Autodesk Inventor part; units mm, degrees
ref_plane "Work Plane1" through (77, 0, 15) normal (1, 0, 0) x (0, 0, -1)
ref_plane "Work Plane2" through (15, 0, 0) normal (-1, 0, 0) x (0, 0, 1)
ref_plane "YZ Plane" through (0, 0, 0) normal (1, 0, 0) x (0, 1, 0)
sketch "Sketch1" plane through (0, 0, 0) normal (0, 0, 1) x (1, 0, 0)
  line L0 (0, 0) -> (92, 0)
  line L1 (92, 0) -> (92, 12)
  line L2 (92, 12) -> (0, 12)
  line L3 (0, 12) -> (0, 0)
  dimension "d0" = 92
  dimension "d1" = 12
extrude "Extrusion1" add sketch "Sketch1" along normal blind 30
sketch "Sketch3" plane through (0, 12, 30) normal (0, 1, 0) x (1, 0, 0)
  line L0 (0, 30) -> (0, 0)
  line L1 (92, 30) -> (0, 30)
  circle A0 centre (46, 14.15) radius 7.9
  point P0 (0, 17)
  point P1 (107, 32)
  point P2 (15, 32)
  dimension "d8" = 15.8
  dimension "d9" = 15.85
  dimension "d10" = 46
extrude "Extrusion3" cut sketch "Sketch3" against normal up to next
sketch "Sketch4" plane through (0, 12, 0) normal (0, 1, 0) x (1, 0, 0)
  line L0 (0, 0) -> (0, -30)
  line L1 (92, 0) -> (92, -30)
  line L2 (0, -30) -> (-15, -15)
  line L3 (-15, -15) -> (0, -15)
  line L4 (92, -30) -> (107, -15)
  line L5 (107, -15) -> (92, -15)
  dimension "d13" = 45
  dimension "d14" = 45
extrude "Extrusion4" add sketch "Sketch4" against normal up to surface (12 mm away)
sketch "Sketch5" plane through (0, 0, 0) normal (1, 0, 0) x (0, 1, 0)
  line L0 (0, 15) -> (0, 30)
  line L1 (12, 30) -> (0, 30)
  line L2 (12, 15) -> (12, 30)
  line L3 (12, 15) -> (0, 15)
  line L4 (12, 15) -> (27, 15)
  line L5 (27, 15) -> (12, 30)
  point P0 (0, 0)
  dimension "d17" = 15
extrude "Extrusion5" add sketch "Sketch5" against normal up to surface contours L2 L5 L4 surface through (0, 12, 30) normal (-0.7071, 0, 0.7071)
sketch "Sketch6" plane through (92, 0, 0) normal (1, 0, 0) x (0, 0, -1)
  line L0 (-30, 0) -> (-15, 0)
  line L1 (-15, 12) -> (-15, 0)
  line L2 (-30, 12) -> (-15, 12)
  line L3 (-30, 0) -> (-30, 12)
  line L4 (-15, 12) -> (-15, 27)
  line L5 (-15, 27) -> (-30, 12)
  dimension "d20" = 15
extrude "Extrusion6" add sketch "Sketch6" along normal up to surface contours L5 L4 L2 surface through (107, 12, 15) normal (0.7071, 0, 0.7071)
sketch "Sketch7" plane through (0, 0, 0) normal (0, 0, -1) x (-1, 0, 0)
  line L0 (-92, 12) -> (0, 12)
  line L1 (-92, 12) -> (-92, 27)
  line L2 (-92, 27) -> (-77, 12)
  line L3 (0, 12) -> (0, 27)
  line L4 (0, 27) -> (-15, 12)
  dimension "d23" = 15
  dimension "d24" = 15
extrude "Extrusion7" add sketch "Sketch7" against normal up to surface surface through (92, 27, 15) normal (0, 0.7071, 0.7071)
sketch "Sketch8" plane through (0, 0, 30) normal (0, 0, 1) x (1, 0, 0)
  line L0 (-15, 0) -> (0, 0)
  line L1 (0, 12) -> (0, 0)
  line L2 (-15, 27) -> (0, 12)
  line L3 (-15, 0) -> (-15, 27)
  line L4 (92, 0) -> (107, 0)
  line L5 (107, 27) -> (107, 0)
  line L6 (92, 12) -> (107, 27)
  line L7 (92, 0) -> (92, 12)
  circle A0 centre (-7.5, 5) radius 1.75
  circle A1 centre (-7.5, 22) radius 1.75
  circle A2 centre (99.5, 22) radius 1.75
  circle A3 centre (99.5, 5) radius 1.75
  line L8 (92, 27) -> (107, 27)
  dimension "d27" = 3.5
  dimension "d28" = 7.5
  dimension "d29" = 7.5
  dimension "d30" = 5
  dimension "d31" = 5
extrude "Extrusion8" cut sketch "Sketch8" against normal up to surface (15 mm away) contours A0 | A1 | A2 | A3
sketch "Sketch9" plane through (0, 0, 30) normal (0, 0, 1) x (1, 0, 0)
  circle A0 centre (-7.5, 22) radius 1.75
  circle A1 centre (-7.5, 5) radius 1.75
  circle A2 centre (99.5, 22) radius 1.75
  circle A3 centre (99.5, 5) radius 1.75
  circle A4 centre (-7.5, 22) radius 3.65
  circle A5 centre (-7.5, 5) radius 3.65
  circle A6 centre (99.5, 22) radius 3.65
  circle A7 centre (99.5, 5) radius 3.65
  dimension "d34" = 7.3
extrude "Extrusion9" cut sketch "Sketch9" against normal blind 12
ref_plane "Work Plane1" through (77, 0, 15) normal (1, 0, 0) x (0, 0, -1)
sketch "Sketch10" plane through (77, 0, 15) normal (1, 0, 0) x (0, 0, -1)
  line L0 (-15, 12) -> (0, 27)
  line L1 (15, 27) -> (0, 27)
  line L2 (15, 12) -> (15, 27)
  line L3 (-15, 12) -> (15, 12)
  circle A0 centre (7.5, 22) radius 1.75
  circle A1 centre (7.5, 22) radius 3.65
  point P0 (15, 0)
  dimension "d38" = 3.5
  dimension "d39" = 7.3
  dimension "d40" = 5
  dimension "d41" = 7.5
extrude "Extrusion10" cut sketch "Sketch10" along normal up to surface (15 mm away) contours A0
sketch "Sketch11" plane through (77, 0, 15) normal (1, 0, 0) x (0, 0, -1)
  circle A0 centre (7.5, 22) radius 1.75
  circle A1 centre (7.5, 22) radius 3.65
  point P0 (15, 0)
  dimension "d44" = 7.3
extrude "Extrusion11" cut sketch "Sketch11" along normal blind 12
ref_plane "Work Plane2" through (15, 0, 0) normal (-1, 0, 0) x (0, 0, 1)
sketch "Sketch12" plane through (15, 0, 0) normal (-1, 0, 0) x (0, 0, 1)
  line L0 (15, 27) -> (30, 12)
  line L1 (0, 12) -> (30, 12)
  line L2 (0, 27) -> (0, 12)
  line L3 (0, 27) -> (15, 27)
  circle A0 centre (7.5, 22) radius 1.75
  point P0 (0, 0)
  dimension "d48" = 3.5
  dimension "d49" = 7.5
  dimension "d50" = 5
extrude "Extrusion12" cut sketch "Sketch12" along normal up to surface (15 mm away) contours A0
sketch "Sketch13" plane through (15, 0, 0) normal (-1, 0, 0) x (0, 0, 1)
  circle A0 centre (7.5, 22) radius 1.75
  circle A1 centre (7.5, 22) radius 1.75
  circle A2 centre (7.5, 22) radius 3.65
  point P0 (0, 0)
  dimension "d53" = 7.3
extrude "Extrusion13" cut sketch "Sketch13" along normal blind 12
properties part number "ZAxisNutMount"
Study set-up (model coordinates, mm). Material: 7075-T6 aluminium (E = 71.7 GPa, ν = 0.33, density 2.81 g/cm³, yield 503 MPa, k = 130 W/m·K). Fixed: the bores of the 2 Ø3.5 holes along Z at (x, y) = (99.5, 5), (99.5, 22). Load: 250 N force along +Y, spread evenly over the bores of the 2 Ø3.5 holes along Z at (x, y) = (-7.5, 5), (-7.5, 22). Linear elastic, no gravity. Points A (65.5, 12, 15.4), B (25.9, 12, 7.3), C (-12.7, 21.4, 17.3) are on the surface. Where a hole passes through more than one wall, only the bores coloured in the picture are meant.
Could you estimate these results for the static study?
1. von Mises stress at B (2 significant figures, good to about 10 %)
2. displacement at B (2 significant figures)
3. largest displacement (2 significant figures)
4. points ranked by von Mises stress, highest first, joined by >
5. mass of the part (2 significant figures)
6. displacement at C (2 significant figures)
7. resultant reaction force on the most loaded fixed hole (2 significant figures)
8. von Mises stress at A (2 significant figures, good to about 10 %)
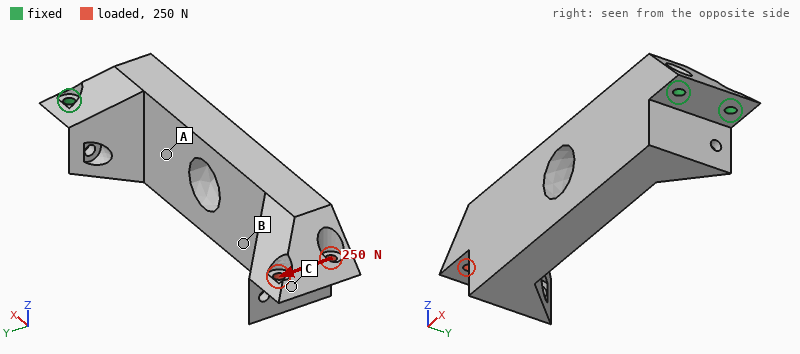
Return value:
12 MPa
0.18 mm
0.40 mm
A > B > C
110 g
0.38 mm
1.5 kN
23 MPa
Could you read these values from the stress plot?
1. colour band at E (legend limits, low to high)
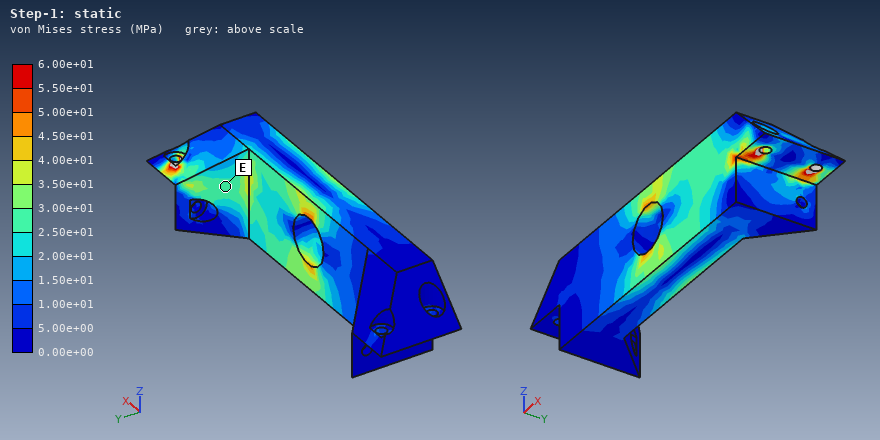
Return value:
2.50e+01 to 3.00e+01 MPa
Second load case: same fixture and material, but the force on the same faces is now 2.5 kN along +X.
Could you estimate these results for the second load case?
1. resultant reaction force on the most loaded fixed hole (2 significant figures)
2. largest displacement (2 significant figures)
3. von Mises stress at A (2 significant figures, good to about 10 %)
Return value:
1.3 kN
0.41 mm
28 MPa
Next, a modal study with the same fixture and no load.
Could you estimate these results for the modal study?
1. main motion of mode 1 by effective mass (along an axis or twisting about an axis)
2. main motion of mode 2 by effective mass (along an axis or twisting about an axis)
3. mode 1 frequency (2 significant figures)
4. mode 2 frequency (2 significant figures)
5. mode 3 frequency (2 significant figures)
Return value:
along Z
along Y
360 Hz
800 Hz
3500 Hz
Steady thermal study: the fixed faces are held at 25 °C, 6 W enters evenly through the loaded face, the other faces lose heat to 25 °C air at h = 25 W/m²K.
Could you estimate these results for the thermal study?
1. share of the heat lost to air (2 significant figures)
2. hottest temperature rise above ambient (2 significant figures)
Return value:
36 %
18 K
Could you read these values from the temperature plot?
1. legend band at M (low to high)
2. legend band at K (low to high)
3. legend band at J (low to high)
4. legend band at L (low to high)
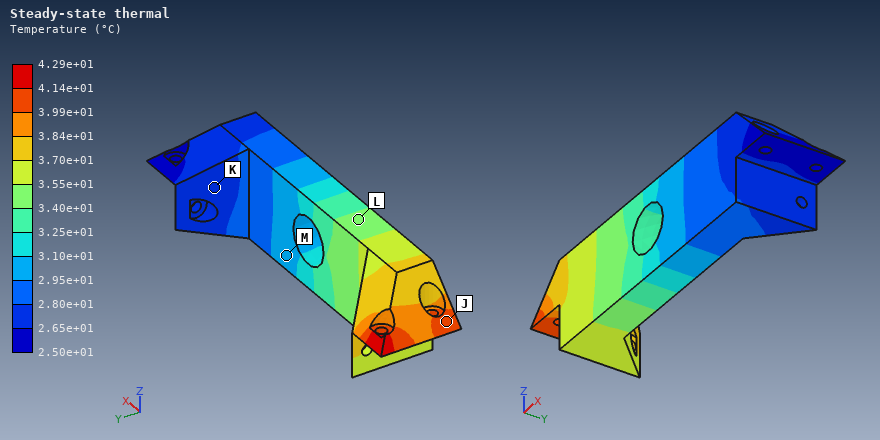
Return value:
2.95e+01 to 3.10e+01 °C
2.65e+01 to 2.80e+01 °C
3.99e+01 to 4.14e+01 °C
3.40e+01 to 3.55e+01 °C
